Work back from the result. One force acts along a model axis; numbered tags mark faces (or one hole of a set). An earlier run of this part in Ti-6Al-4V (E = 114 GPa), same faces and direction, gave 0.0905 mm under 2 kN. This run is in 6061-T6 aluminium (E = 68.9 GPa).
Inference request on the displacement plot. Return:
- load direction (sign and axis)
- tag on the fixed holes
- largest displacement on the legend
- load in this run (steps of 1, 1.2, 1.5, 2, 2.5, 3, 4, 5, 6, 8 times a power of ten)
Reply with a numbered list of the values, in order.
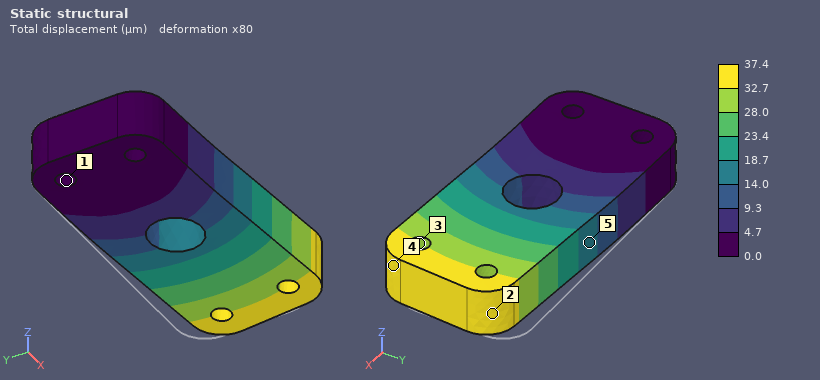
1. -Y
2. 1
3. 37.4 µm
4. 500 N
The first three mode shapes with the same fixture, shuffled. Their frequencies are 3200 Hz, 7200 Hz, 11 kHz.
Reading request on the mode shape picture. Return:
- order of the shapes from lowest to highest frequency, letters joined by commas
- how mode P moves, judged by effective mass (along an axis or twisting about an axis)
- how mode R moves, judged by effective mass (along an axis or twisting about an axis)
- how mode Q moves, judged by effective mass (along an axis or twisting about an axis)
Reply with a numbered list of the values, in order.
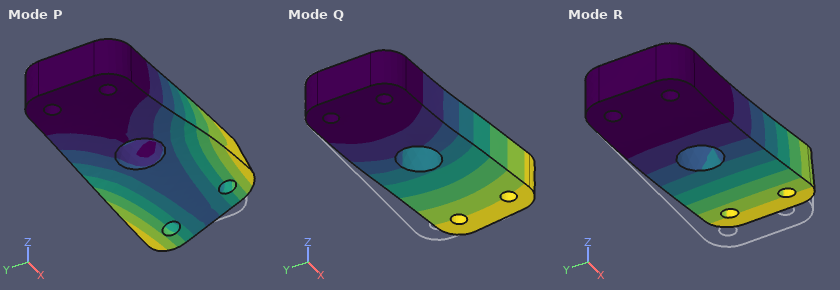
1. R, Q, P
2. twisting about X
3. along Z
4. along Y
